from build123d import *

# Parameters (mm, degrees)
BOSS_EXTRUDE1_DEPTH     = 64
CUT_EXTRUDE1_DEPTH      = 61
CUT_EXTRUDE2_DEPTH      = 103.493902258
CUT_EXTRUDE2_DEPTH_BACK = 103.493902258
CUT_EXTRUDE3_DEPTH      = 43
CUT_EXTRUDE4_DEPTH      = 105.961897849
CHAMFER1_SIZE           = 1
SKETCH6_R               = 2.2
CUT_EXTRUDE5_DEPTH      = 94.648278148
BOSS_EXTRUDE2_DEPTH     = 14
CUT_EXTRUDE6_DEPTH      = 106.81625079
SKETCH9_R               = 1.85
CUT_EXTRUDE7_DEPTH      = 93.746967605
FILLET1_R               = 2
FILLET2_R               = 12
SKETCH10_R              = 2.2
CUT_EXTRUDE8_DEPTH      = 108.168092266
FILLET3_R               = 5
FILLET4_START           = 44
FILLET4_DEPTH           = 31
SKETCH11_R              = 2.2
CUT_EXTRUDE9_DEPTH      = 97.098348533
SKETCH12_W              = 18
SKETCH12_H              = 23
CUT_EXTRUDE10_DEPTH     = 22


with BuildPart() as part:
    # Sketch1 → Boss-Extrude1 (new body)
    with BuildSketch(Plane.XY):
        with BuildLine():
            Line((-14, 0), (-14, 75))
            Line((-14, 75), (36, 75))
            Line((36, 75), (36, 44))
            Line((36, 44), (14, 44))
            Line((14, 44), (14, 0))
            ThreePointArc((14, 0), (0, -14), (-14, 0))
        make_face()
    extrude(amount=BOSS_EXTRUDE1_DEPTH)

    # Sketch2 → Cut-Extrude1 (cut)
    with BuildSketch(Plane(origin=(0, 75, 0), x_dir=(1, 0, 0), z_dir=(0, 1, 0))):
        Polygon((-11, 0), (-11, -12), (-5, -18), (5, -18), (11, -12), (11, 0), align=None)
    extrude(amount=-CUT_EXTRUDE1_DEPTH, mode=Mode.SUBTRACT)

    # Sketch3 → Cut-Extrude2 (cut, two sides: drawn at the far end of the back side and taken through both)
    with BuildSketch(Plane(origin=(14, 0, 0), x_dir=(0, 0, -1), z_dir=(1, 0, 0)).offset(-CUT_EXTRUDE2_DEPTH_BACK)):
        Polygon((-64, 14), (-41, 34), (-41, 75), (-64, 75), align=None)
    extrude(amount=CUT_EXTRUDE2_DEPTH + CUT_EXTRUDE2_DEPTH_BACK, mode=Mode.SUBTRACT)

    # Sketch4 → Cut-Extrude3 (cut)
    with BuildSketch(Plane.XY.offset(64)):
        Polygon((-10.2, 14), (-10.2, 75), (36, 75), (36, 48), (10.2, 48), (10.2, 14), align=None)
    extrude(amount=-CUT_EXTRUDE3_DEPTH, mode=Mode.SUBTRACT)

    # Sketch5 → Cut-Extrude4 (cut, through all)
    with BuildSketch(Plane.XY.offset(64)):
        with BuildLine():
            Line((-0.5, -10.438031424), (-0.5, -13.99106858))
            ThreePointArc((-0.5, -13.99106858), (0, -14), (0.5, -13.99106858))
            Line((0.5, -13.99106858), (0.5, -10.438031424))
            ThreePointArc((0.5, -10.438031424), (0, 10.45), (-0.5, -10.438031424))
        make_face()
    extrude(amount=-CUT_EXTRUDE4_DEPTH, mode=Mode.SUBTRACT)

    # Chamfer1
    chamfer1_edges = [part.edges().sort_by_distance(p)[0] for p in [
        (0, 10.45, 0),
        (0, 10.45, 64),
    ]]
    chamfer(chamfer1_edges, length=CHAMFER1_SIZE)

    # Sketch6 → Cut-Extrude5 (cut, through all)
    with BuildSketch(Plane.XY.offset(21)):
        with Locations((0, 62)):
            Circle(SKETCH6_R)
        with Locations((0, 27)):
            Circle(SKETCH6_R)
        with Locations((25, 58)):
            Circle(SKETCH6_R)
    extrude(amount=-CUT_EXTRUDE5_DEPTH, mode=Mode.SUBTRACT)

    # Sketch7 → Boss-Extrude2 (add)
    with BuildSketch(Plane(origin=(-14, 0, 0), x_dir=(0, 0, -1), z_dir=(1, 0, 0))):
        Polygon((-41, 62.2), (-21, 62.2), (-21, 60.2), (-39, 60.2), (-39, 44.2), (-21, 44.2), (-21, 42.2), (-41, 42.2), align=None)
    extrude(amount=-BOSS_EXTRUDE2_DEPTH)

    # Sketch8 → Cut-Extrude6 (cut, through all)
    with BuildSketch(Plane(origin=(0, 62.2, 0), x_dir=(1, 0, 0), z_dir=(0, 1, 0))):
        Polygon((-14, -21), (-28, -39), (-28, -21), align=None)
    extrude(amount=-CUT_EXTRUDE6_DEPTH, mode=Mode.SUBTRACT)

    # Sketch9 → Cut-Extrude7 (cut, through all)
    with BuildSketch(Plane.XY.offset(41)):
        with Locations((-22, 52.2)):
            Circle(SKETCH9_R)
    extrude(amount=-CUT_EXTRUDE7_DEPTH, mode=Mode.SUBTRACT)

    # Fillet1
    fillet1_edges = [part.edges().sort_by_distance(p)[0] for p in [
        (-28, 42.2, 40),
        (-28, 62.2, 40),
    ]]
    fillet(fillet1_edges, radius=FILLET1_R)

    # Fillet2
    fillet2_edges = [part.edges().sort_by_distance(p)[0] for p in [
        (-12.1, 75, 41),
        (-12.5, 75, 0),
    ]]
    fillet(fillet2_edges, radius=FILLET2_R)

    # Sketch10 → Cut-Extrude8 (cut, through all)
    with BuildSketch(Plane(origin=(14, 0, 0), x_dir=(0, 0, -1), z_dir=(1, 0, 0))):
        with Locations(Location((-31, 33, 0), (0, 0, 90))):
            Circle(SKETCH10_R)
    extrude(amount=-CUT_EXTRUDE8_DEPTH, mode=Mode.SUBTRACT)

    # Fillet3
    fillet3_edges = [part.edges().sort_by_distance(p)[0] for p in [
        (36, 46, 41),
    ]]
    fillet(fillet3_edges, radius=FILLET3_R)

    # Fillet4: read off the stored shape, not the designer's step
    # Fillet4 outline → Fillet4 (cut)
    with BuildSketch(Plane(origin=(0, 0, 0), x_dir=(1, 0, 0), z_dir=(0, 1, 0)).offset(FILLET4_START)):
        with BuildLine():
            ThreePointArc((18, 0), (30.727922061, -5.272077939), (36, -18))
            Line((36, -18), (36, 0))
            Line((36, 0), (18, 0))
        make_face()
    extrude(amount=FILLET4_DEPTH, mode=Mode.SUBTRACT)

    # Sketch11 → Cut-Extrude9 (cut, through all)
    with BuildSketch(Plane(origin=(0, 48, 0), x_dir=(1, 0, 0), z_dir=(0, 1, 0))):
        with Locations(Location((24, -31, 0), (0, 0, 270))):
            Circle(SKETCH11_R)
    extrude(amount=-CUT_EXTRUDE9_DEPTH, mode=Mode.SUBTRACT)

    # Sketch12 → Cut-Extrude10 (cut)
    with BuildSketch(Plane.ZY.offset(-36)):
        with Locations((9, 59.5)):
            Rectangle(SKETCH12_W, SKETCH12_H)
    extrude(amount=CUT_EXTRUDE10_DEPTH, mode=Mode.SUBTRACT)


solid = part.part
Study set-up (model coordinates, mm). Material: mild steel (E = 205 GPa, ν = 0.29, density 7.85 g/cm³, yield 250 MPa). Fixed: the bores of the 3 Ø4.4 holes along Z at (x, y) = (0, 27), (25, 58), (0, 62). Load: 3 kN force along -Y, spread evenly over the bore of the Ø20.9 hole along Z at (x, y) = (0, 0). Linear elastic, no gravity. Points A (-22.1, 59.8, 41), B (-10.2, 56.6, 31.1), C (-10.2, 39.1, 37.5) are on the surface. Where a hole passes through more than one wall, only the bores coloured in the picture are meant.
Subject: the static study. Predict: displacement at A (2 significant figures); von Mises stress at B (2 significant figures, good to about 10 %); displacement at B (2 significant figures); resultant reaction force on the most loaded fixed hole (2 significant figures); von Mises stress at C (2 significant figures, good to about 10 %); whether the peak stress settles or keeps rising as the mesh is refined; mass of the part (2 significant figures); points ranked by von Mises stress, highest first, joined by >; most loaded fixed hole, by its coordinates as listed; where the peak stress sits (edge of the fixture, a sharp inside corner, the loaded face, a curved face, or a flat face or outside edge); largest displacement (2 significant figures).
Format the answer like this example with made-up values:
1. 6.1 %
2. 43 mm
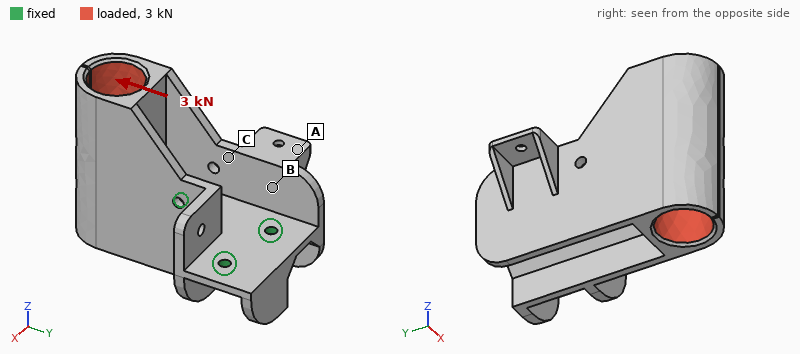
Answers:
1. 27 µm
2. 12 MPa
3. 14 µm
4. 2.3 kN
5. 17 MPa
6. keeps rising
7. 410 g
8. C > B > A
9. (0, 27)
10. edge of the fixture
11. 55 µm
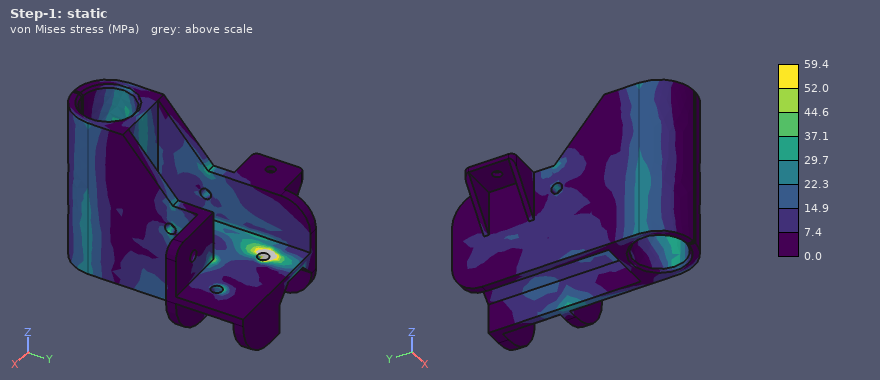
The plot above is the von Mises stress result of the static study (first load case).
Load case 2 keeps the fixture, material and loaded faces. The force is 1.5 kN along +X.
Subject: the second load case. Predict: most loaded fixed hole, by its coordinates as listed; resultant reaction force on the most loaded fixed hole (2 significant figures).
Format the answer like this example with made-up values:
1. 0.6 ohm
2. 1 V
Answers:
1. (0, 27)
2. 2.3 kN
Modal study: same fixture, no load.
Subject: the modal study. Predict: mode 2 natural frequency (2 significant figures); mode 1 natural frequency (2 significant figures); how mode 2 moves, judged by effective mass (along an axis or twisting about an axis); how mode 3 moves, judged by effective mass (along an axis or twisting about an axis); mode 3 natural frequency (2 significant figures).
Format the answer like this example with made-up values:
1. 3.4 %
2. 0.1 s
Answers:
1. 2400 Hz
2. 1500 Hz
3. along Z
4. along Z
5. 3600 Hz
